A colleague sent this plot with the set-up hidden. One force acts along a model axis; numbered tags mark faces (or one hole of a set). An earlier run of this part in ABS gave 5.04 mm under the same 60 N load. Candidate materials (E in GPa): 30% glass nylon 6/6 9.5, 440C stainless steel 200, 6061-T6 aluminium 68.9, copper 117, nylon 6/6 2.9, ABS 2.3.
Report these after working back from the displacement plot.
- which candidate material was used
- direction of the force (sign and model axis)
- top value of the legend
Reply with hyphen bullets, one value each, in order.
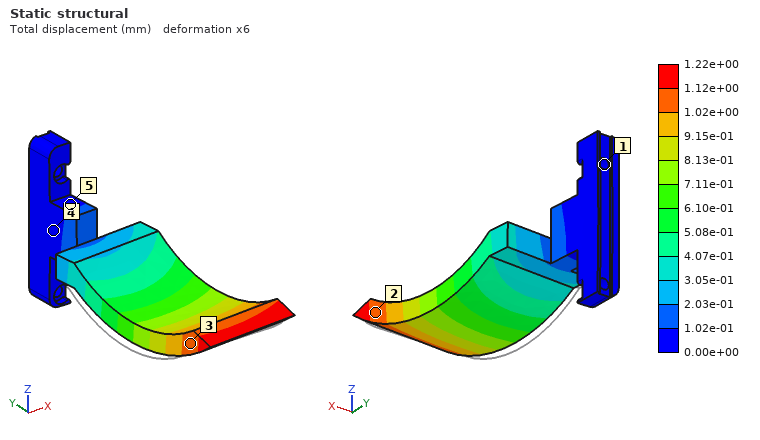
- 30% glass nylon 6/6
- +X
- 1.22e+00 mm
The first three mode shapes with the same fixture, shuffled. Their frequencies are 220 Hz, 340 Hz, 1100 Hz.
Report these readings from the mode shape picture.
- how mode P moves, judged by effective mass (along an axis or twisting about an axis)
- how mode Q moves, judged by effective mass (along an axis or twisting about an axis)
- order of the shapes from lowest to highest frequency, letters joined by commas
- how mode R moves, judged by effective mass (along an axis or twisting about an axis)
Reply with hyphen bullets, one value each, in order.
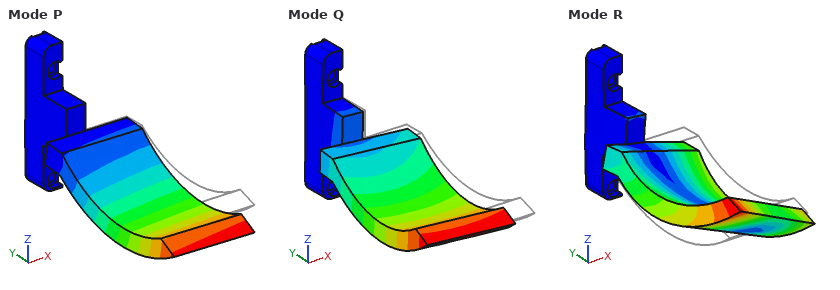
- along Z
- along X
- Q, P, R
- twisting about Y
